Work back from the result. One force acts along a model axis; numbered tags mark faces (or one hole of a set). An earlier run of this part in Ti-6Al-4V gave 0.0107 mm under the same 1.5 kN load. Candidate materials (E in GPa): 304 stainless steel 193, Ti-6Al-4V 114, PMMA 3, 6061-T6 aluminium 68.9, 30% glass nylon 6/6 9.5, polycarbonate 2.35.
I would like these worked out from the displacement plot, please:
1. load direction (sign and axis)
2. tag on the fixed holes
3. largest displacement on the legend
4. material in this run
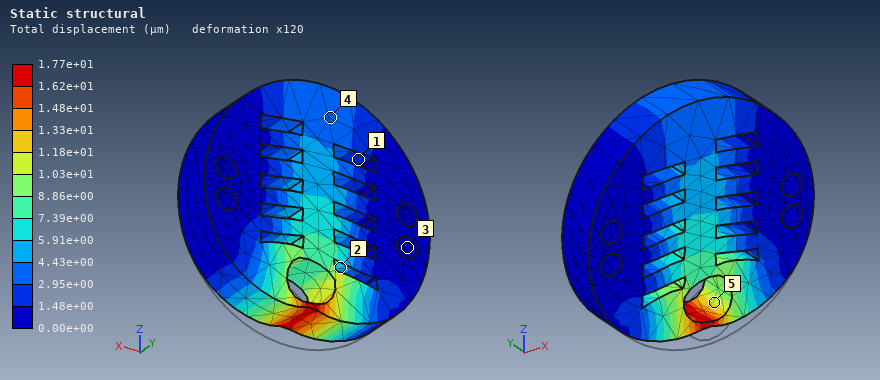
+Z
3
1.77e+01 µm
6061-T6 aluminium
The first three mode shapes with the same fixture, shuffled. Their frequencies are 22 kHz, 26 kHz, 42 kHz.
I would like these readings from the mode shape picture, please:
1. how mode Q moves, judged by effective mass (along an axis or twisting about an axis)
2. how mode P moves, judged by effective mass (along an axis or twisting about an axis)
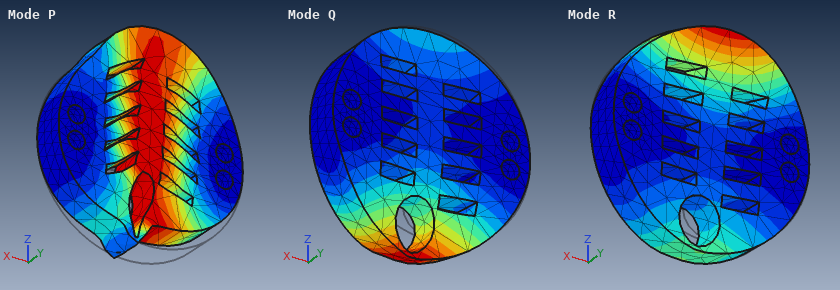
along Y
along Z
